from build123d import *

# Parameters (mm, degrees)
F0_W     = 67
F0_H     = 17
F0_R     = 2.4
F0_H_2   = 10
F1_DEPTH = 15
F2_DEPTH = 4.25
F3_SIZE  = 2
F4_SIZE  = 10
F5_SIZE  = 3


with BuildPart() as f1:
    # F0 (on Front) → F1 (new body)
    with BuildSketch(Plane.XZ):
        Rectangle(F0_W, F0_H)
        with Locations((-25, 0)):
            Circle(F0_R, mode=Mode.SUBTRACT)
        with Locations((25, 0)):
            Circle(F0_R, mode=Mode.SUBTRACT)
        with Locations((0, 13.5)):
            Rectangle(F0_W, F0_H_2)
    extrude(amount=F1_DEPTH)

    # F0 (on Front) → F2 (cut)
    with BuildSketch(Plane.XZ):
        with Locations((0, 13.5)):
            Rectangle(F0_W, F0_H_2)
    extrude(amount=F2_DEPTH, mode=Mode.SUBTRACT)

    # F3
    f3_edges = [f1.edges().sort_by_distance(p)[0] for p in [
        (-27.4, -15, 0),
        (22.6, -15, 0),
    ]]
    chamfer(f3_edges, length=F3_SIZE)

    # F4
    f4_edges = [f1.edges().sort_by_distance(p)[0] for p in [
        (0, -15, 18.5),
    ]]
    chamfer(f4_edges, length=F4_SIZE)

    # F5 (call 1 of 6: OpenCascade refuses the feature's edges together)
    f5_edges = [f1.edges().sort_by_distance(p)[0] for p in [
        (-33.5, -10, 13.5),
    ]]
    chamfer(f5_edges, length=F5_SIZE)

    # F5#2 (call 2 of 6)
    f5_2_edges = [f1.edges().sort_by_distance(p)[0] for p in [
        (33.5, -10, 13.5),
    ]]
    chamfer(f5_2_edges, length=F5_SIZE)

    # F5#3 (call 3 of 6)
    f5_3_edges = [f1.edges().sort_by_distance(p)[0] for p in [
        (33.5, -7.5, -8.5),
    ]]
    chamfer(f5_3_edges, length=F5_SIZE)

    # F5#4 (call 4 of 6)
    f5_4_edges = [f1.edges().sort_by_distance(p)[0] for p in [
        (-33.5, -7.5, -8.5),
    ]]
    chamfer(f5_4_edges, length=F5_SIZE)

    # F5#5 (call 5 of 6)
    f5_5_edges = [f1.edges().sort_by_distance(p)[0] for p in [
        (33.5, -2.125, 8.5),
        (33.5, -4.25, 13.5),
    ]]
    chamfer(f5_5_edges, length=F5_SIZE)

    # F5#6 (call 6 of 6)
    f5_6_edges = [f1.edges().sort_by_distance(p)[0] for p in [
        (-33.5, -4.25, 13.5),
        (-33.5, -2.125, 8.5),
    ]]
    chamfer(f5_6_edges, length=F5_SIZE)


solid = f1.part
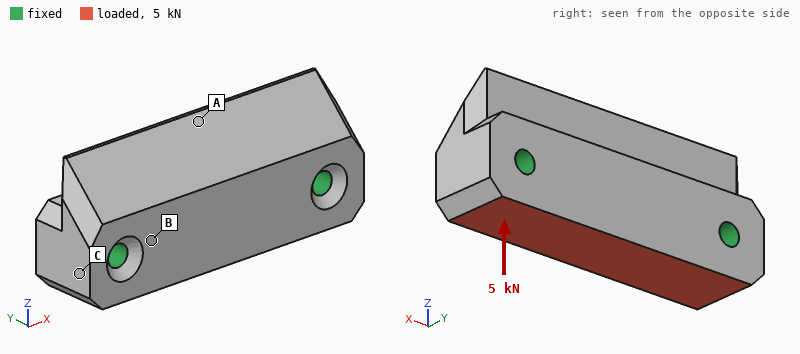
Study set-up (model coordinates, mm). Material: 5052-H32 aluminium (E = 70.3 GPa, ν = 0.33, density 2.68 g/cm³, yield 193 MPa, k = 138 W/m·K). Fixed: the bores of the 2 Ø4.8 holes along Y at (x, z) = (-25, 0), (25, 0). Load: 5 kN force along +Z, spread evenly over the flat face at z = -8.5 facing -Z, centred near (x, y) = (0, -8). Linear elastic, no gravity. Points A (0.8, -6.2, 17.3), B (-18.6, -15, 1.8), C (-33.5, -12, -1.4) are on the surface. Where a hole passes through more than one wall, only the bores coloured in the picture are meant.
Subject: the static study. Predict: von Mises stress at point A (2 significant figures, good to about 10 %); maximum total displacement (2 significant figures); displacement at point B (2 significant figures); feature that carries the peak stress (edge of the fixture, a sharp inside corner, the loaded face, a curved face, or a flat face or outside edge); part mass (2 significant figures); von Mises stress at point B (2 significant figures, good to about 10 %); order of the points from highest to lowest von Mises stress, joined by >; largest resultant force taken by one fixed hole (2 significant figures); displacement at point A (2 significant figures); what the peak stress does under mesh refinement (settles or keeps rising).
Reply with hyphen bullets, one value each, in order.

- 19 MPa
- 8.0 µm
- 3.0 µm
- edge of the fixture
- 53 g
- 11 MPa
- A > B > C
- 2.5 kN
- 6.3 µm
- keeps rising
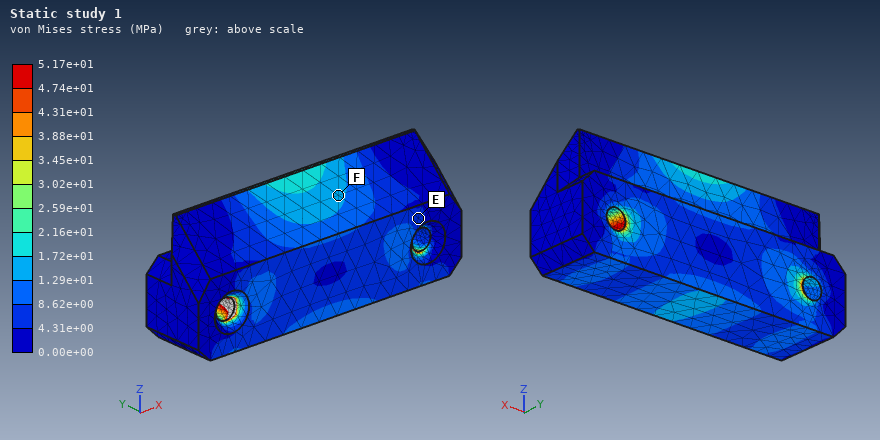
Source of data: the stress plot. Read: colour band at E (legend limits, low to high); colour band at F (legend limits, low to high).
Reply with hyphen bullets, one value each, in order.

- 4.31e+00 to 8.62e+00 MPa
- 1.29e+01 to 1.72e+01 MPa
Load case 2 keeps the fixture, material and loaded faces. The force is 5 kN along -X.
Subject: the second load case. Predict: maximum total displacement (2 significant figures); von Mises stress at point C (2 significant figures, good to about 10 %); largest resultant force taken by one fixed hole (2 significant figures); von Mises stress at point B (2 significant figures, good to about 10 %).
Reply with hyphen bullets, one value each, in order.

- 3.1 µm
- 9.0 MPa
- 2.6 kN
- 5.8 MPa
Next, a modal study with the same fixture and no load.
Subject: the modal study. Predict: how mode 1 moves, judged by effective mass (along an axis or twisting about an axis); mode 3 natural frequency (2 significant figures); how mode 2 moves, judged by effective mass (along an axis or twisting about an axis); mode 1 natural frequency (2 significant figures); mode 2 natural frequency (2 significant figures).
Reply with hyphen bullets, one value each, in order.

- along Y
- 23 kHz
- along Z
- 18 kHz
- 20 kHz
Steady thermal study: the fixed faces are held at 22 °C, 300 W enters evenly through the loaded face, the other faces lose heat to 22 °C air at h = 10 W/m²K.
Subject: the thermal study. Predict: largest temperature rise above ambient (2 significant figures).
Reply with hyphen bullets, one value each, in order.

- 56 K
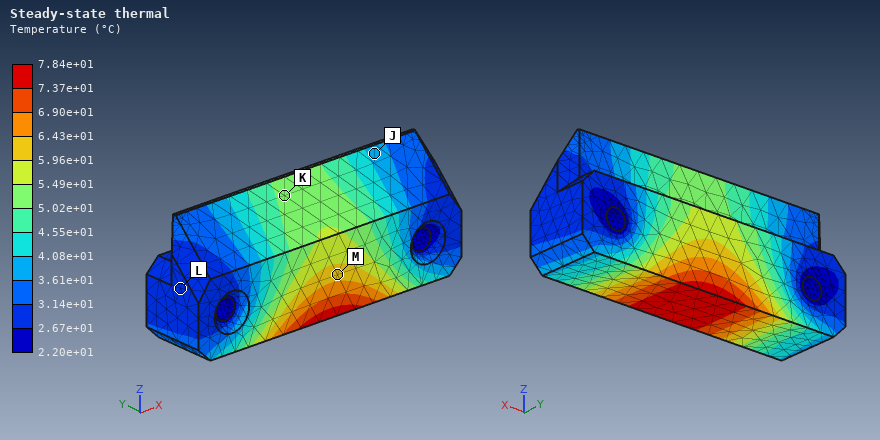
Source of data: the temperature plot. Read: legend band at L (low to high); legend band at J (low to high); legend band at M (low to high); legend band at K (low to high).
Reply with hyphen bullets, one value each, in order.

- 2.67e+01 to 3.14e+01 °C
- 3.61e+01 to 4.08e+01 °C
- 5.96e+01 to 6.43e+01 °C
- 5.02e+01 to 5.49e+01 °C
